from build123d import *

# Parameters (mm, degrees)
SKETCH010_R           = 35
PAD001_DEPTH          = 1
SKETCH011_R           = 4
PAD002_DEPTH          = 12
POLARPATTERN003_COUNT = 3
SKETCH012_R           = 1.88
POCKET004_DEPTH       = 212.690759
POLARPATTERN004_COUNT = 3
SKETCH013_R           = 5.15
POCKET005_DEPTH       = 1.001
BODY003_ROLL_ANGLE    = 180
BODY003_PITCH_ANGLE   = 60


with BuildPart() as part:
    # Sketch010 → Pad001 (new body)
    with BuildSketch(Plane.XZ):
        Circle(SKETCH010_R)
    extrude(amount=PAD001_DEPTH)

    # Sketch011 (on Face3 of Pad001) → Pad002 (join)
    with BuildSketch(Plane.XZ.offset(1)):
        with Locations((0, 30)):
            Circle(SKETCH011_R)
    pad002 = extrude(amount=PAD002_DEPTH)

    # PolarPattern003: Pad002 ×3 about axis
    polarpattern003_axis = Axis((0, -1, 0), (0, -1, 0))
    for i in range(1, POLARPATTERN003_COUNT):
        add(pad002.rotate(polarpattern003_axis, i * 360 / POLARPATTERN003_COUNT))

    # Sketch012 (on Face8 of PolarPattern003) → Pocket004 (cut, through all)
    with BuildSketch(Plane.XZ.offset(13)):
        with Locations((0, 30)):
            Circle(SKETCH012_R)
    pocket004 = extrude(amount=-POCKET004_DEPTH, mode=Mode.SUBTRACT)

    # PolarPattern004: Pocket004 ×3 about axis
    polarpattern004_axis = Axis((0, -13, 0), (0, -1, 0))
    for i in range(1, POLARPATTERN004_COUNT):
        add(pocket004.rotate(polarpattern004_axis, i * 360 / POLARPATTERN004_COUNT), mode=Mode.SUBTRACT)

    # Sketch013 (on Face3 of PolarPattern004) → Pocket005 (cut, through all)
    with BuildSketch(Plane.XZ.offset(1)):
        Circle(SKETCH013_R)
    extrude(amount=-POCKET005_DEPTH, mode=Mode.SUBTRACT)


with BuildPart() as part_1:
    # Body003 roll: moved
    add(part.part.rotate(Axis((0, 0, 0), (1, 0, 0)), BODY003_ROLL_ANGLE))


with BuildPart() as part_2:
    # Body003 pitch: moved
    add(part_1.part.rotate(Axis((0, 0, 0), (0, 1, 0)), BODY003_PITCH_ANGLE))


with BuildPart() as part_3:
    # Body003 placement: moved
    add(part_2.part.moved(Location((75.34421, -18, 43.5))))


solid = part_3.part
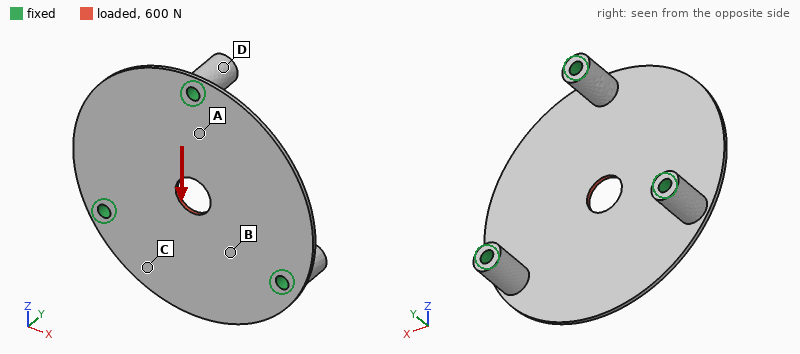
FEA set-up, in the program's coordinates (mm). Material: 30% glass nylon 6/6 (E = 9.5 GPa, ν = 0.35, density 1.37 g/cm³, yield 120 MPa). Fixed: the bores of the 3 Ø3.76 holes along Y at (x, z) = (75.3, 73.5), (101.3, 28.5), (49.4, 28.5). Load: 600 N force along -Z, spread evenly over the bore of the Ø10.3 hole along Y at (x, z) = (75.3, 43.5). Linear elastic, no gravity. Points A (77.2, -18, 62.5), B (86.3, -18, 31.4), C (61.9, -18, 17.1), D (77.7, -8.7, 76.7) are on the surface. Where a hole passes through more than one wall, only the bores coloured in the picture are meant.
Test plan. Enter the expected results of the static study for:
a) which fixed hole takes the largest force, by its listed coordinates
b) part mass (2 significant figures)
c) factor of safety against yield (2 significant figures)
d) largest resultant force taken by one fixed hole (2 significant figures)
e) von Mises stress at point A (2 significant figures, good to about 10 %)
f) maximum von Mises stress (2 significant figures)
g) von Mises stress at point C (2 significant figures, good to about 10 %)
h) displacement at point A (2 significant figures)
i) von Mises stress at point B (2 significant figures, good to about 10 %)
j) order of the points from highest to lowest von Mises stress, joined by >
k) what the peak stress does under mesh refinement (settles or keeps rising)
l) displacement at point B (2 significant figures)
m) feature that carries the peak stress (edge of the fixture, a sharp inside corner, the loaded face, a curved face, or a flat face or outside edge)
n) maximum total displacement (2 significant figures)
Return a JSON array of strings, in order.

["(75.3, 73.5)", "7.0 g", "3.6", "230 N", "16 MPa", "33 MPa", "6.5 MPa", "19 µm", "8.7 MPa", "A > B > C > D", "settles", "30 µm", "the loaded face", "54 µm"]
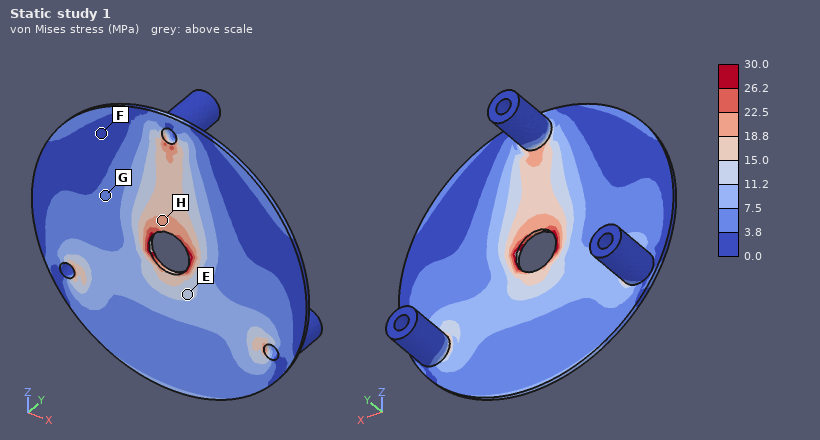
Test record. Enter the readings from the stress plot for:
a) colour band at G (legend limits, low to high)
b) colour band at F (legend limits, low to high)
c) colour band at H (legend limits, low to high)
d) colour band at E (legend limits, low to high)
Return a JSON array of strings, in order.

["3.8 to 7.5 MPa", "0.0 to 3.8 MPa", "18.8 to 22.5 MPa", "11.2 to 15.0 MPa"]
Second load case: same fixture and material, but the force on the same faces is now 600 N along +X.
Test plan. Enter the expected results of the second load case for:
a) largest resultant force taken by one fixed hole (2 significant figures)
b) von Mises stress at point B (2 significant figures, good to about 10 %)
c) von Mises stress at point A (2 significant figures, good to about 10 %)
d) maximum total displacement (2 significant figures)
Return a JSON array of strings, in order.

["210 N", "11 MPa", "3.5 MPa", "53 µm"]
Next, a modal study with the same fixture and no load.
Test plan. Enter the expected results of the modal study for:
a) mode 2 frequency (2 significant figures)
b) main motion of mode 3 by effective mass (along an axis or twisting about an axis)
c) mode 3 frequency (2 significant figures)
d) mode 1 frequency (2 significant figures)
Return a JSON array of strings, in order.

["870 Hz", "along Y", "930 Hz", "870 Hz"]
